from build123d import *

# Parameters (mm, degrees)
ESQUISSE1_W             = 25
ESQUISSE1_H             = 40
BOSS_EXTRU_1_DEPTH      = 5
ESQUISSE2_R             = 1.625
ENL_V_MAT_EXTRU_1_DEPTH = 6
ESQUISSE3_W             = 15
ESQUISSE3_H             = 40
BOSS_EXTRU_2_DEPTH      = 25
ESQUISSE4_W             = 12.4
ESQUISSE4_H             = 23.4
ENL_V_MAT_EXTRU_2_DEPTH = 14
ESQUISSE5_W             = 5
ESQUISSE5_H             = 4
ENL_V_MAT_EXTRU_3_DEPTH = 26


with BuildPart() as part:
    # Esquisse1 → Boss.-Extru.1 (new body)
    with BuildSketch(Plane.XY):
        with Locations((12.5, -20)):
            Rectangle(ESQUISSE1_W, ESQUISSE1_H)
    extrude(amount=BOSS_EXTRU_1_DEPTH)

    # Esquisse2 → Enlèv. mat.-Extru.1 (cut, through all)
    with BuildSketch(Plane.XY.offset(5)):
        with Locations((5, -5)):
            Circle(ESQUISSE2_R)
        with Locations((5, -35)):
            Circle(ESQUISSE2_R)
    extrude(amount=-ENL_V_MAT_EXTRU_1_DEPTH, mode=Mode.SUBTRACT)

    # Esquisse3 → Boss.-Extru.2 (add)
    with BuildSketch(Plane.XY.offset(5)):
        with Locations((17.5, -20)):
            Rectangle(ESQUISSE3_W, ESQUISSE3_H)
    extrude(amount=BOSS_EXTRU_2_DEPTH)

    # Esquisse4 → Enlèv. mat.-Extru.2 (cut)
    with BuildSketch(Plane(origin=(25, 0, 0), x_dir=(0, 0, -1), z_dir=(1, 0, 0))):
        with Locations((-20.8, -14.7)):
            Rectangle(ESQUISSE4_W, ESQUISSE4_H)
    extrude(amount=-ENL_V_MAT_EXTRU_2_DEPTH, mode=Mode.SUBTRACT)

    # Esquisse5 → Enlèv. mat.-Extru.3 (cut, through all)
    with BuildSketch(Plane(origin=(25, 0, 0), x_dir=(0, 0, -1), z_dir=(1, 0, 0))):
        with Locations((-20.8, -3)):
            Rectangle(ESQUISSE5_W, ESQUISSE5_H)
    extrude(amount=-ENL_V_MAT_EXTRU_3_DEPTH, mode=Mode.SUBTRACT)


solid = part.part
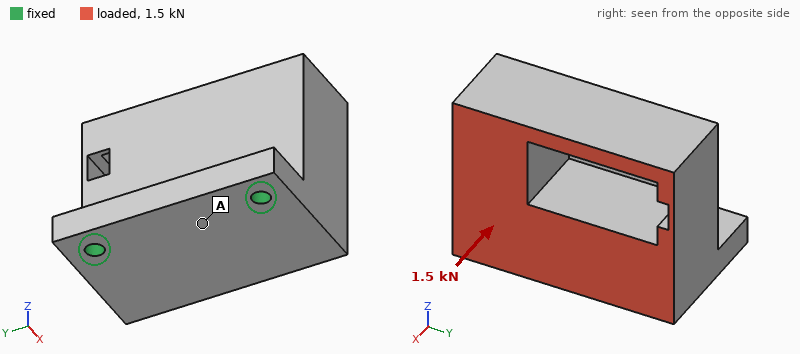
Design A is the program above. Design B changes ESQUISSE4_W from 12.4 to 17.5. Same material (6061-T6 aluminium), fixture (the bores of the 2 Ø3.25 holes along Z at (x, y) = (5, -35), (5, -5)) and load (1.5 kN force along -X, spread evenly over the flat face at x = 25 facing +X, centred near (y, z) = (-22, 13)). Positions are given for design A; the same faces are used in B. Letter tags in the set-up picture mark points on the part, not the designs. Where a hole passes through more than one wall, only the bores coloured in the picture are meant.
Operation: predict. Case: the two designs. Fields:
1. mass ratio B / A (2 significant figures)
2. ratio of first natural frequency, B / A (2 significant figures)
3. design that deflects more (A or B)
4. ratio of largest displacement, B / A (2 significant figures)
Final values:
0.89
1.1
A
0.91
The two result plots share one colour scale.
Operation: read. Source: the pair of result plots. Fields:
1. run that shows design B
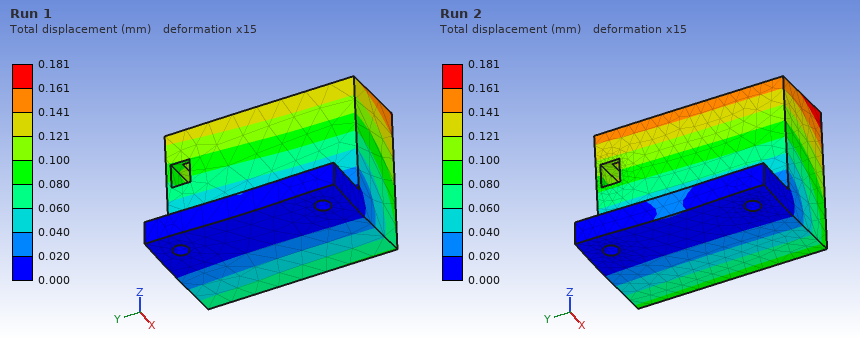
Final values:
Run 1
